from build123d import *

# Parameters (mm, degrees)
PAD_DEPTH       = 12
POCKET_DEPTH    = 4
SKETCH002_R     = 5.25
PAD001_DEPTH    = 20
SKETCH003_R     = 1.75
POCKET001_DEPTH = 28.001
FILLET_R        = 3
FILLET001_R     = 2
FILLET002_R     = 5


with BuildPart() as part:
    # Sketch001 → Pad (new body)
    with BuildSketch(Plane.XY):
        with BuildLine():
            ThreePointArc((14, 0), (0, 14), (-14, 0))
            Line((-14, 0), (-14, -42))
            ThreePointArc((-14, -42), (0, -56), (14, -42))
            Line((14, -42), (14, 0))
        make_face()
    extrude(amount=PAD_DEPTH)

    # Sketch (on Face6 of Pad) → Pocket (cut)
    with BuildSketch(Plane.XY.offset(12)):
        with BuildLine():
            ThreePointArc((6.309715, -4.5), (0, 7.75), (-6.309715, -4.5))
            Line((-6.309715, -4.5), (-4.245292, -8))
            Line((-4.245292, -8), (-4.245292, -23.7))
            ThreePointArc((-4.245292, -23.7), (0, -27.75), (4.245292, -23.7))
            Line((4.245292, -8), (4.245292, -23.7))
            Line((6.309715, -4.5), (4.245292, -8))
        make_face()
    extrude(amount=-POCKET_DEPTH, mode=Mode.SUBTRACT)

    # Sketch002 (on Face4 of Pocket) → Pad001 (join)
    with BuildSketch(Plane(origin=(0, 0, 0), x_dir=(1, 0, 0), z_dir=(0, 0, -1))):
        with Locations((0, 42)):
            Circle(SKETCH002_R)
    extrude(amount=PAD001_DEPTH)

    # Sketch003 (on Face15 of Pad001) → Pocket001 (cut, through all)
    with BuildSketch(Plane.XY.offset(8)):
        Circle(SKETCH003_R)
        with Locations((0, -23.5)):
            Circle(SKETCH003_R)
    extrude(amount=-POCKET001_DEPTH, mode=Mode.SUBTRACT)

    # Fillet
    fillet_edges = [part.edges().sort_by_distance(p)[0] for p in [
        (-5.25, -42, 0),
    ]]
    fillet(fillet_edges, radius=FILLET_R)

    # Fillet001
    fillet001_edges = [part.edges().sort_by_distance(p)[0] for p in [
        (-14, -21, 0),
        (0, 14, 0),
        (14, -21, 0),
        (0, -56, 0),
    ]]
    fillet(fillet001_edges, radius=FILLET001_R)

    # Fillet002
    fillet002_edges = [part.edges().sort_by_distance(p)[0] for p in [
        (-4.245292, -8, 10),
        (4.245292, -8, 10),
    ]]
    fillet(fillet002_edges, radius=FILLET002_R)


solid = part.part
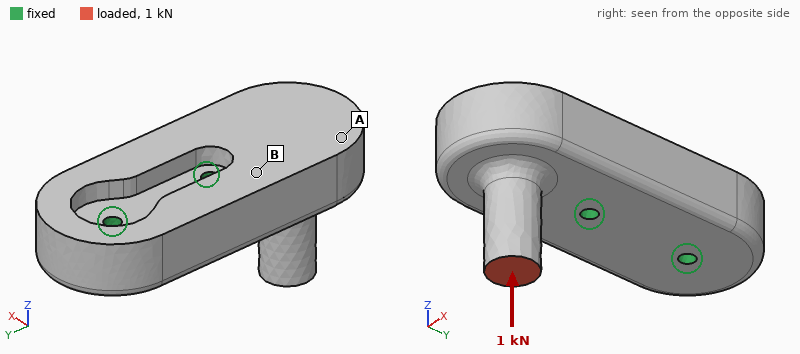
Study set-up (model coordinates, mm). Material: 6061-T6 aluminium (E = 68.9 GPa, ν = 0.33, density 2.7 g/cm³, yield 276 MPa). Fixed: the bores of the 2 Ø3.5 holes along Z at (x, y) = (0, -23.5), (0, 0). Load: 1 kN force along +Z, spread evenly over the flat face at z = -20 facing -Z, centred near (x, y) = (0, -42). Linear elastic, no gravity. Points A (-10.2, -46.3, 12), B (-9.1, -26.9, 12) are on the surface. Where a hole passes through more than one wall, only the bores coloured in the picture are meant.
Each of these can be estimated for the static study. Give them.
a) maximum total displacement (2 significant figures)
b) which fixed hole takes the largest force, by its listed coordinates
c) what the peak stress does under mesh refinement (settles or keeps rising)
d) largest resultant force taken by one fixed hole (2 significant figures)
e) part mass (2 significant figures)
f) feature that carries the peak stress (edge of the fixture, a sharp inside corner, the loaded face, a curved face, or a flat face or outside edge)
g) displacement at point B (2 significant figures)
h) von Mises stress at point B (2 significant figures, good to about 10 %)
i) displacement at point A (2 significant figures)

43 µm
(0, -23.5)
keeps rising
1.5 kN
58 g
edge of the fixture
7.1 µm
22 MPa
27 µm
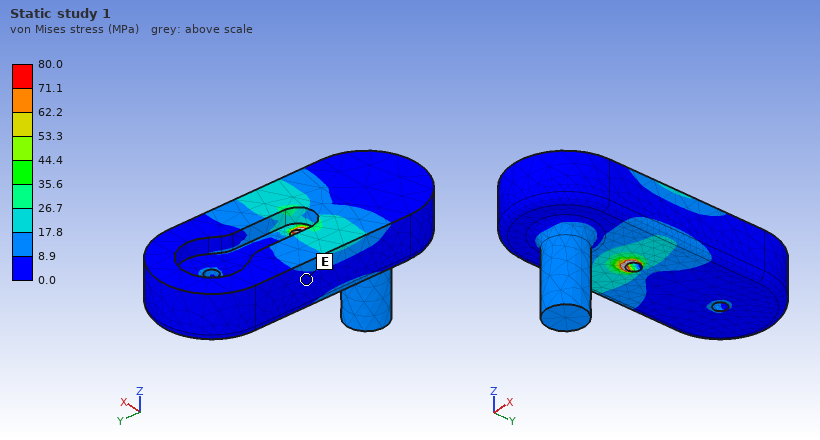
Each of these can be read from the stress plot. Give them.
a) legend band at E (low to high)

0.0 to 8.9 MPa
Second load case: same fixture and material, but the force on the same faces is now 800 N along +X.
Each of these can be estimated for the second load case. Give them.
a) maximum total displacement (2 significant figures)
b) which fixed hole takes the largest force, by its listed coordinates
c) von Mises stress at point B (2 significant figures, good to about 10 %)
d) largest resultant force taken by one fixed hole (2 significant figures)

0.12 mm
(0, -23.5)
16 MPa
1.3 kN
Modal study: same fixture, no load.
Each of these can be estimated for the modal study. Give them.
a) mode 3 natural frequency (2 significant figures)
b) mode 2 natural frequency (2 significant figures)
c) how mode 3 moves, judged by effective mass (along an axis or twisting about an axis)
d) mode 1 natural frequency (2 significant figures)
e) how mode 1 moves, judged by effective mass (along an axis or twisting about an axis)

10 kHz
8200 Hz
along X
5900 Hz
along Z
